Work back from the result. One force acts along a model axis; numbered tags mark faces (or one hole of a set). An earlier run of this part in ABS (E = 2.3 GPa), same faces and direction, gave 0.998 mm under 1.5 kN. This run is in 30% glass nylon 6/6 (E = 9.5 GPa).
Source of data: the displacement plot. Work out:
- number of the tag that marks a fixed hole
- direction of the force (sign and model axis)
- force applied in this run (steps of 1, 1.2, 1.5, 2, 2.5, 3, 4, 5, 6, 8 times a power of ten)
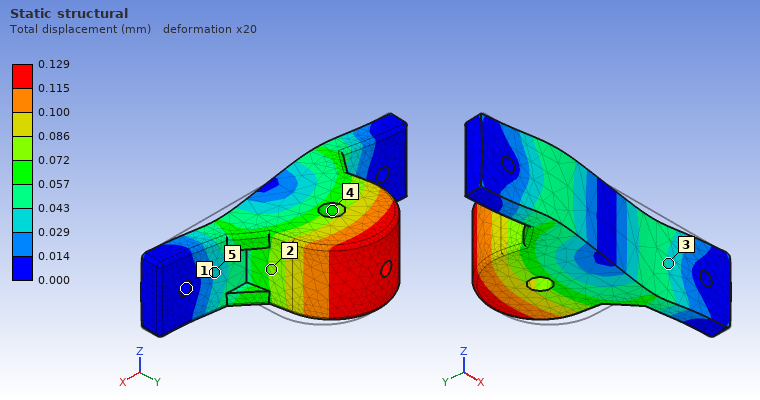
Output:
1
-X
800 N
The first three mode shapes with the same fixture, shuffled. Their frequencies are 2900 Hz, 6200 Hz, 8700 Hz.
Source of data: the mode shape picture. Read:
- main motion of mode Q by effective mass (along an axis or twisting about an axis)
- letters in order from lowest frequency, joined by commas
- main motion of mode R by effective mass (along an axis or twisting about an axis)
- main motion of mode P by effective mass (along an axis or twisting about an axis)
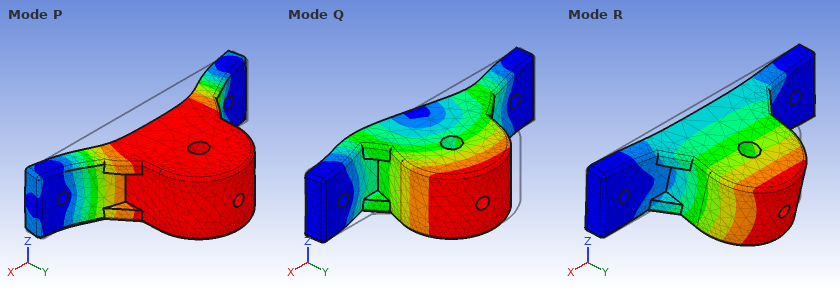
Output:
along X
R, P, Q
along Z
along Y
